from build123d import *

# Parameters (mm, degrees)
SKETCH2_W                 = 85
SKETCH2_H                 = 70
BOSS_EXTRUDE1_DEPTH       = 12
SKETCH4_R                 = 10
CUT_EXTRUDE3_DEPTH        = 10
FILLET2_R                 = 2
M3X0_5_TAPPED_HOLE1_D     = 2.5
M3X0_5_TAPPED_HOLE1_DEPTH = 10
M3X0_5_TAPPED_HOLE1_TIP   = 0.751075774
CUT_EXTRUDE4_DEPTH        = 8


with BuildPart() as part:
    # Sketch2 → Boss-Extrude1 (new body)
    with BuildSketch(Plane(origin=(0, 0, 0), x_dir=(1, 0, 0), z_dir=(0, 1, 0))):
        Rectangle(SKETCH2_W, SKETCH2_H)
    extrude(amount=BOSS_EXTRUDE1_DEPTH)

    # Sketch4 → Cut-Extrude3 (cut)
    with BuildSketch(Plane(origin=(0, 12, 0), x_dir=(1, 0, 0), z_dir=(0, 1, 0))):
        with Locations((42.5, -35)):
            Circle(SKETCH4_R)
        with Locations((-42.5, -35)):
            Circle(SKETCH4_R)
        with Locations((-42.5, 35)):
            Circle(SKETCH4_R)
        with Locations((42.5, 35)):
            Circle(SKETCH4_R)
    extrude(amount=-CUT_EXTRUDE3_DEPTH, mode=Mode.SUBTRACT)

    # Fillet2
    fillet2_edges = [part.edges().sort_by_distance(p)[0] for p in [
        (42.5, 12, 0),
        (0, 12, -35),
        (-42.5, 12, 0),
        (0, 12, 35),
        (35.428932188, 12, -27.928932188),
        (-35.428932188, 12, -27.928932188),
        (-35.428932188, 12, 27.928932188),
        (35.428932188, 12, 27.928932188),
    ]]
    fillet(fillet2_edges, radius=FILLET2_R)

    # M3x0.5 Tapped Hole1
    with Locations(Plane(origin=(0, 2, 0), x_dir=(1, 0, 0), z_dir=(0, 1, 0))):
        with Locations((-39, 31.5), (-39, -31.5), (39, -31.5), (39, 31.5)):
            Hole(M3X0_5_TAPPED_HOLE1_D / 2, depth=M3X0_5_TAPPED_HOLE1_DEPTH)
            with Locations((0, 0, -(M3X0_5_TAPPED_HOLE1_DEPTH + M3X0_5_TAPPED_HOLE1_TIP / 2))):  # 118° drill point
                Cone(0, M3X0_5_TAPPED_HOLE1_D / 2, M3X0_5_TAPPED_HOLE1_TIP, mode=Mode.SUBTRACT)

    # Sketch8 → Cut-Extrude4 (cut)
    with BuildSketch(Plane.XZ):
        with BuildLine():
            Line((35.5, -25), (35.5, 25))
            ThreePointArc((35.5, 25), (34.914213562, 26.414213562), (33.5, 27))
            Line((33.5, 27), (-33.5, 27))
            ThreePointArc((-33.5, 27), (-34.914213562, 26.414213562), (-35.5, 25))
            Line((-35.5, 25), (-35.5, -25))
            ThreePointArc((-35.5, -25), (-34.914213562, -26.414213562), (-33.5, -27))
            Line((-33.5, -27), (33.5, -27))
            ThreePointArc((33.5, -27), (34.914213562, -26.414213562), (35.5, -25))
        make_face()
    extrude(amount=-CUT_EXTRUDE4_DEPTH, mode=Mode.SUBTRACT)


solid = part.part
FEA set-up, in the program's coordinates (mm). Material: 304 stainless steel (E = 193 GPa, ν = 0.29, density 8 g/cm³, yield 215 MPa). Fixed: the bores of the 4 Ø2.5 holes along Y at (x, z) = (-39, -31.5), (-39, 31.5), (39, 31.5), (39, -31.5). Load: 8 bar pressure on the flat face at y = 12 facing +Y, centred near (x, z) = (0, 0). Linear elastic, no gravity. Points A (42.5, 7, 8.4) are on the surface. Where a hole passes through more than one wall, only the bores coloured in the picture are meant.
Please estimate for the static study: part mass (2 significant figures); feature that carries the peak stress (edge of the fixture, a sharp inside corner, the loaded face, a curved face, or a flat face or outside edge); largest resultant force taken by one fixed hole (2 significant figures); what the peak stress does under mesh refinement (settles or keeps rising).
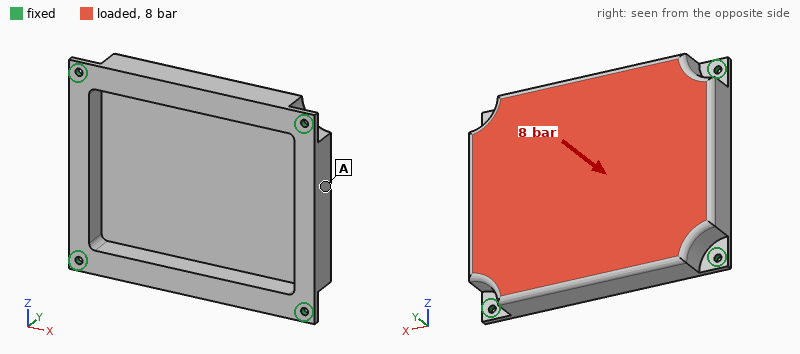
300 g
edge of the fixture
1.7 kN
keeps rising
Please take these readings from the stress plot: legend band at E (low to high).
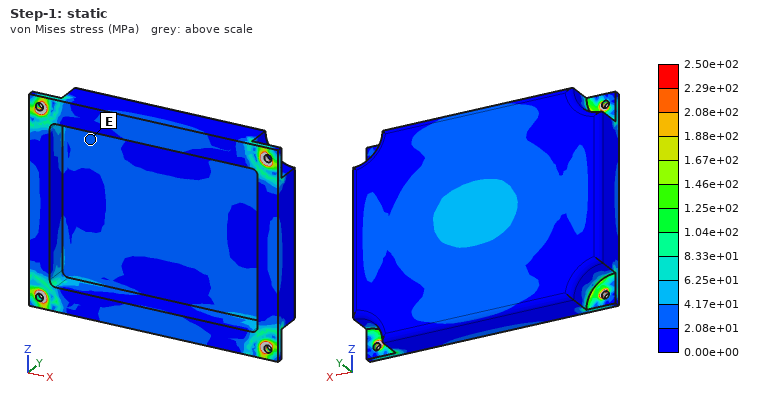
2.08e+01 to 4.17e+01 MPa
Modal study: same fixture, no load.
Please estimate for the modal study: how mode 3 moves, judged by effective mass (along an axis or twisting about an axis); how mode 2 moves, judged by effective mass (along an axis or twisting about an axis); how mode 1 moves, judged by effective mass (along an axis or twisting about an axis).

twisting about Z
twisting about X
along Y
